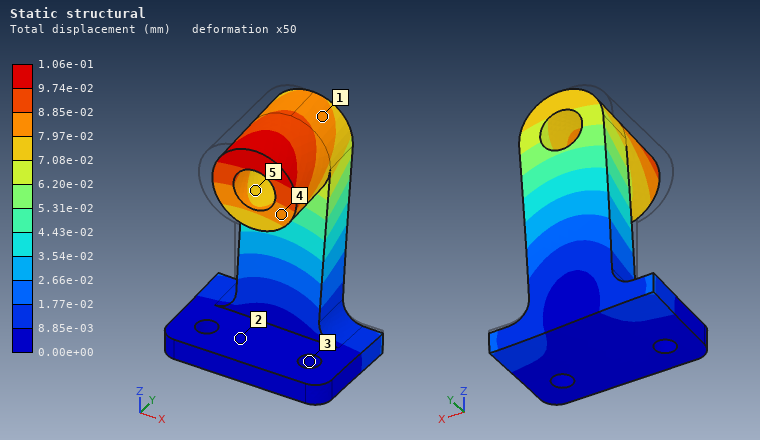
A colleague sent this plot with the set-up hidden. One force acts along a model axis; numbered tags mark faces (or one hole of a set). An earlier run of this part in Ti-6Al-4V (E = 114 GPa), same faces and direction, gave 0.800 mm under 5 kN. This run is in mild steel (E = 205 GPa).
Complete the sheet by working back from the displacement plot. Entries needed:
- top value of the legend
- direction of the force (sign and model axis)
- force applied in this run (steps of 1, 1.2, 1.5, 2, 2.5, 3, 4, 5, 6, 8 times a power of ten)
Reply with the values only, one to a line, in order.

1.06e-01 mm
+X
1.2 kN
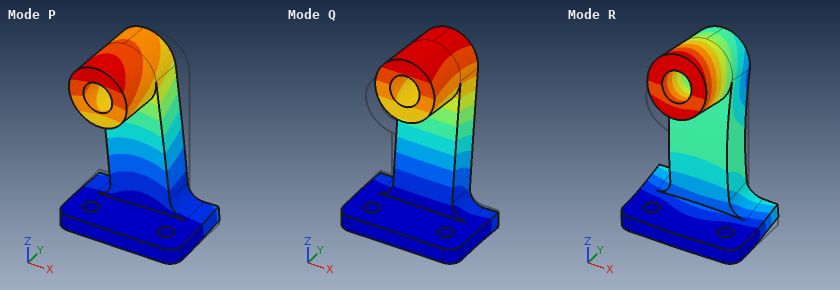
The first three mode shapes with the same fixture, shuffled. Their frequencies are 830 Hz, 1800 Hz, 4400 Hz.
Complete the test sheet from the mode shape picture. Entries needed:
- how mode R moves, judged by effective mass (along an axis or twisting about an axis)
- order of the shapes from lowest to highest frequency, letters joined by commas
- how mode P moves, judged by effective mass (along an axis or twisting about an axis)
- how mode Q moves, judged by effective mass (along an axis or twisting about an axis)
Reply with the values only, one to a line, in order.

along Z
Q, P, R
along X
along Y
